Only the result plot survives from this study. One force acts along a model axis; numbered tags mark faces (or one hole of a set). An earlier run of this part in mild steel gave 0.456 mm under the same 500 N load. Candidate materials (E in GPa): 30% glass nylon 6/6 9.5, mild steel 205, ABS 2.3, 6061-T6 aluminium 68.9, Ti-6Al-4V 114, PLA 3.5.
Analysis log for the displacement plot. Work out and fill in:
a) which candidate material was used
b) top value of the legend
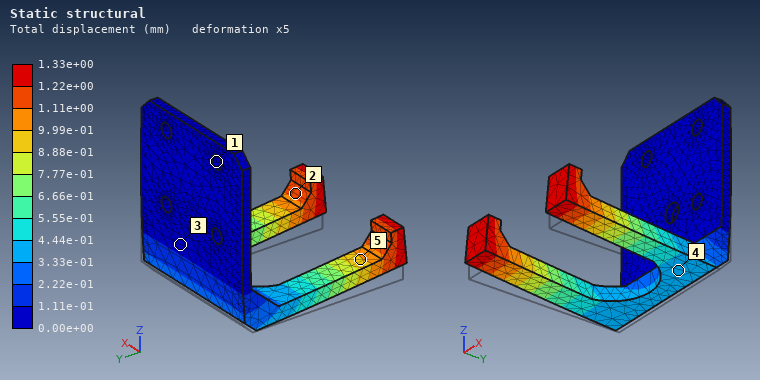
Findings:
6061-T6 aluminium
1.33e+00 mm
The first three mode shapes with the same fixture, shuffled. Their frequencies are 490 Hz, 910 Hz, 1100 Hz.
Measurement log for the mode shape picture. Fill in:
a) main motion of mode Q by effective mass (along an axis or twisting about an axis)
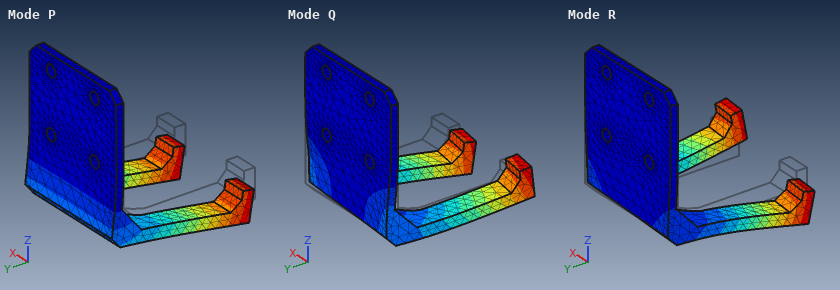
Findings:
along X
